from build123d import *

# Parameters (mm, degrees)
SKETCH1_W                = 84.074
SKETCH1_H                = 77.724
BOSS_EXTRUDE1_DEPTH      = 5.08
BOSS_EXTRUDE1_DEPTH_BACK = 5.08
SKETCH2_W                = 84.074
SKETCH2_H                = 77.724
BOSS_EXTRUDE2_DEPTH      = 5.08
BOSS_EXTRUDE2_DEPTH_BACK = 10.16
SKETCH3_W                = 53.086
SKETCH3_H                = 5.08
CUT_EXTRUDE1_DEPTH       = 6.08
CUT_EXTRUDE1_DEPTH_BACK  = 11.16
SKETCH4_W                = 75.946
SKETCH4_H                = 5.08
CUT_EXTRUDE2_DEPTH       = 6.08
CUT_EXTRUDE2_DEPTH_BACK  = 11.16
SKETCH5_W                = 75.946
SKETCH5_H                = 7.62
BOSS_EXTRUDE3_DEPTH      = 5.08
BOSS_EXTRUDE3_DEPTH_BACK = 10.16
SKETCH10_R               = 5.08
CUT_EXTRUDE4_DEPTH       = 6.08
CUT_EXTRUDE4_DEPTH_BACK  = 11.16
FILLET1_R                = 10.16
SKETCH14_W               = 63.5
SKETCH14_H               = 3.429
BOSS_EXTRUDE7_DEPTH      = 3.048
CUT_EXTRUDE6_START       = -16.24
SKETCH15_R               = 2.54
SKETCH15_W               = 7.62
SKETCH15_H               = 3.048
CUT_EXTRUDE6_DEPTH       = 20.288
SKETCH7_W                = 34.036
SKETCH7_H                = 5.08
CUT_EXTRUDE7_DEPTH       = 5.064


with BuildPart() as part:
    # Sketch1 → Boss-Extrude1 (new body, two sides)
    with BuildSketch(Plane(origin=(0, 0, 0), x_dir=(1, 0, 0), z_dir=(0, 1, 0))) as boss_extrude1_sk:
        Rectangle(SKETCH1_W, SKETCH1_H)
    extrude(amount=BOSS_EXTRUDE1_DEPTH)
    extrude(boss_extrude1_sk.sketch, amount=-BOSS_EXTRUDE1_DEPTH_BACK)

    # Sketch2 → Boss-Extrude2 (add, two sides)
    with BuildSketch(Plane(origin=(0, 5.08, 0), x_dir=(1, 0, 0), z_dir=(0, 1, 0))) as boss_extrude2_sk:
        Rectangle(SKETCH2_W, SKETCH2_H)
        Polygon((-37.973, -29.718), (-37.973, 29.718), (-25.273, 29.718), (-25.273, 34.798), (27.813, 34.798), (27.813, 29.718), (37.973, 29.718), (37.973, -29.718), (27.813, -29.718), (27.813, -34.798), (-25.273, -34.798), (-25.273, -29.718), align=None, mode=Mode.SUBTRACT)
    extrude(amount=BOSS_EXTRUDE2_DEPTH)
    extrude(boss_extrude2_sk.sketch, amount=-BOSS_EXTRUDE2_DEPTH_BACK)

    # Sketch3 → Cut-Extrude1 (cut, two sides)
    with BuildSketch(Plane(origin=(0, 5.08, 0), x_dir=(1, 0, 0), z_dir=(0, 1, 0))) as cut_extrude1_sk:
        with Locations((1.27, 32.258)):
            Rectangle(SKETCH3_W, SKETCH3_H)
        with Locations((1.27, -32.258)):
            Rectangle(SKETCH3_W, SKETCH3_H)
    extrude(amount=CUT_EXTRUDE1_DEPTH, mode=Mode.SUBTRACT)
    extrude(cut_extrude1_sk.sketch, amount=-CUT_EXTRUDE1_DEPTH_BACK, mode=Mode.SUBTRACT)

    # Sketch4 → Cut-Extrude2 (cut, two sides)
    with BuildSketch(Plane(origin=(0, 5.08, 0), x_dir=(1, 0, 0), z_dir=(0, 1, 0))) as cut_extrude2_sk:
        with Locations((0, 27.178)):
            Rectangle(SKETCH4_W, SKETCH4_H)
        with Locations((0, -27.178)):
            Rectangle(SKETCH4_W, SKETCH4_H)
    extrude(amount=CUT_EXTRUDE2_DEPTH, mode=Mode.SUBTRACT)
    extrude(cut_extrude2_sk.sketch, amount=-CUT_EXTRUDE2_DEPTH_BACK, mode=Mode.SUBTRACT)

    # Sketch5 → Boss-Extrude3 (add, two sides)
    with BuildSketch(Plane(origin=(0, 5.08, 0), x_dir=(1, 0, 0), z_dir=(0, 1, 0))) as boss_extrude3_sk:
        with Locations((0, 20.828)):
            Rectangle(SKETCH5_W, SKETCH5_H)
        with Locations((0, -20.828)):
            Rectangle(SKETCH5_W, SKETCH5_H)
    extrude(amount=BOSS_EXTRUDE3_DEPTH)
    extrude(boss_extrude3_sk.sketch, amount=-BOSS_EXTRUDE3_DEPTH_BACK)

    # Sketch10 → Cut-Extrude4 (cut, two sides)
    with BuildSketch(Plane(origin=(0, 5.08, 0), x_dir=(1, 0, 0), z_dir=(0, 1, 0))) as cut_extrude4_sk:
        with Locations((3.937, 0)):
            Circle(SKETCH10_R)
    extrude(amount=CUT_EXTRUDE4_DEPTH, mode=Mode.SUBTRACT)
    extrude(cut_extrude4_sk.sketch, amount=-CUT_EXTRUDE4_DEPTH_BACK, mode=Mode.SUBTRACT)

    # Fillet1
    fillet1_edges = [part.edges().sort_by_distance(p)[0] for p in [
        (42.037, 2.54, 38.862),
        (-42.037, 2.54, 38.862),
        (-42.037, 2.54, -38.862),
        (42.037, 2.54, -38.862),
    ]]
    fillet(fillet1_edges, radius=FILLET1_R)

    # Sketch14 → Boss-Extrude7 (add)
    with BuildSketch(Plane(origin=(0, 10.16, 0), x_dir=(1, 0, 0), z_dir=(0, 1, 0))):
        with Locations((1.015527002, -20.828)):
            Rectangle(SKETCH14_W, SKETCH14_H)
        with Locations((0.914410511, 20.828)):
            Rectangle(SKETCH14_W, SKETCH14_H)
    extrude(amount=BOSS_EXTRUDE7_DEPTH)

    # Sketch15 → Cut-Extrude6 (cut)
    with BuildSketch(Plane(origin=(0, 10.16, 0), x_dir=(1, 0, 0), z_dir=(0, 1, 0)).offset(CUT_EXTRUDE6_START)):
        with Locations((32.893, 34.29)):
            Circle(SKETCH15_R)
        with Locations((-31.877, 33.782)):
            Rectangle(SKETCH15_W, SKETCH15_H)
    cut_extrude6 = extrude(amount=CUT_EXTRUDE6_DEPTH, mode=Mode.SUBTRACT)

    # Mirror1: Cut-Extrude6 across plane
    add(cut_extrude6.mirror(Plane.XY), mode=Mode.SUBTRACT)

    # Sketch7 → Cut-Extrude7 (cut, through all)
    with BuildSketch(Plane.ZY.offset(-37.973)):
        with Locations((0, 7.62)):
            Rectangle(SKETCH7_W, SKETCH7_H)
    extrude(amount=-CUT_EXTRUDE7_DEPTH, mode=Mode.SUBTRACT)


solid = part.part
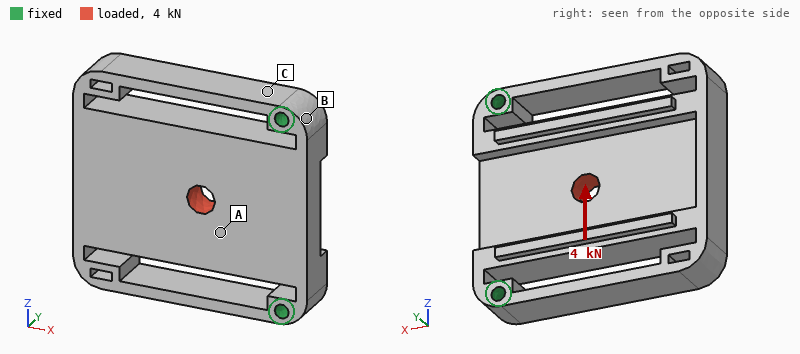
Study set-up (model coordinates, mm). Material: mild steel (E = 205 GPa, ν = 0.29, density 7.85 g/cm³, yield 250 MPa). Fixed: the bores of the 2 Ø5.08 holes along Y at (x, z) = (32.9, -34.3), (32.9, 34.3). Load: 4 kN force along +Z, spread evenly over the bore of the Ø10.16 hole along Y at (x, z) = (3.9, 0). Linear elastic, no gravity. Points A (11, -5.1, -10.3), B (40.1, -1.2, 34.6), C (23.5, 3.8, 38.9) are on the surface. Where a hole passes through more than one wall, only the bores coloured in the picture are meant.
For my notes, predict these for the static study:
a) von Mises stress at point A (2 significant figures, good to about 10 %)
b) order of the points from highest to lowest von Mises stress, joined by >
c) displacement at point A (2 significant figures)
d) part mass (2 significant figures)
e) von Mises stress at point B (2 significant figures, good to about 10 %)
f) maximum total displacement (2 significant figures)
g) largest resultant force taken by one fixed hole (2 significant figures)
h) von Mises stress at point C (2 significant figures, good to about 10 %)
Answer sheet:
13 MPa
B > C > A
24 µm
500 g
74 MPa
58 µm
3.0 kN
44 MPa
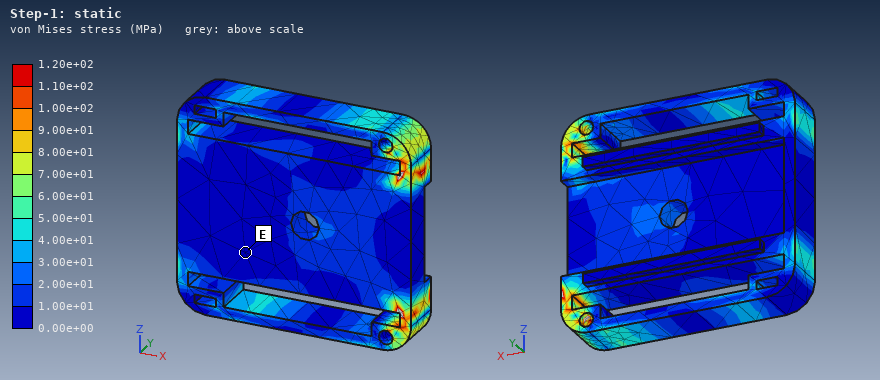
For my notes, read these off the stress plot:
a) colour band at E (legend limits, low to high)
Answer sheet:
0.00e+00 to 1.00e+01 MPa
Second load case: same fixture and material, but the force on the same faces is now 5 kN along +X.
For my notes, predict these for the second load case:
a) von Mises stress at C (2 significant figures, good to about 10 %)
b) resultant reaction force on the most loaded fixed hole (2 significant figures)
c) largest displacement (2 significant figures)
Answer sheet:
22 MPa
2.5 kN
36 µm
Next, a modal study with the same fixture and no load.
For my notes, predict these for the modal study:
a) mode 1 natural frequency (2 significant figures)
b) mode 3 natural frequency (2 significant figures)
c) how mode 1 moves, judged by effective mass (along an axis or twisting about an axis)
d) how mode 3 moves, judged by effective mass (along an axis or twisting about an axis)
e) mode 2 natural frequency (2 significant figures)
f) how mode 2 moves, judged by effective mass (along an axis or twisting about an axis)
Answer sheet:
910 Hz
2900 Hz
along Y
twisting about X
2000 Hz
along Z
